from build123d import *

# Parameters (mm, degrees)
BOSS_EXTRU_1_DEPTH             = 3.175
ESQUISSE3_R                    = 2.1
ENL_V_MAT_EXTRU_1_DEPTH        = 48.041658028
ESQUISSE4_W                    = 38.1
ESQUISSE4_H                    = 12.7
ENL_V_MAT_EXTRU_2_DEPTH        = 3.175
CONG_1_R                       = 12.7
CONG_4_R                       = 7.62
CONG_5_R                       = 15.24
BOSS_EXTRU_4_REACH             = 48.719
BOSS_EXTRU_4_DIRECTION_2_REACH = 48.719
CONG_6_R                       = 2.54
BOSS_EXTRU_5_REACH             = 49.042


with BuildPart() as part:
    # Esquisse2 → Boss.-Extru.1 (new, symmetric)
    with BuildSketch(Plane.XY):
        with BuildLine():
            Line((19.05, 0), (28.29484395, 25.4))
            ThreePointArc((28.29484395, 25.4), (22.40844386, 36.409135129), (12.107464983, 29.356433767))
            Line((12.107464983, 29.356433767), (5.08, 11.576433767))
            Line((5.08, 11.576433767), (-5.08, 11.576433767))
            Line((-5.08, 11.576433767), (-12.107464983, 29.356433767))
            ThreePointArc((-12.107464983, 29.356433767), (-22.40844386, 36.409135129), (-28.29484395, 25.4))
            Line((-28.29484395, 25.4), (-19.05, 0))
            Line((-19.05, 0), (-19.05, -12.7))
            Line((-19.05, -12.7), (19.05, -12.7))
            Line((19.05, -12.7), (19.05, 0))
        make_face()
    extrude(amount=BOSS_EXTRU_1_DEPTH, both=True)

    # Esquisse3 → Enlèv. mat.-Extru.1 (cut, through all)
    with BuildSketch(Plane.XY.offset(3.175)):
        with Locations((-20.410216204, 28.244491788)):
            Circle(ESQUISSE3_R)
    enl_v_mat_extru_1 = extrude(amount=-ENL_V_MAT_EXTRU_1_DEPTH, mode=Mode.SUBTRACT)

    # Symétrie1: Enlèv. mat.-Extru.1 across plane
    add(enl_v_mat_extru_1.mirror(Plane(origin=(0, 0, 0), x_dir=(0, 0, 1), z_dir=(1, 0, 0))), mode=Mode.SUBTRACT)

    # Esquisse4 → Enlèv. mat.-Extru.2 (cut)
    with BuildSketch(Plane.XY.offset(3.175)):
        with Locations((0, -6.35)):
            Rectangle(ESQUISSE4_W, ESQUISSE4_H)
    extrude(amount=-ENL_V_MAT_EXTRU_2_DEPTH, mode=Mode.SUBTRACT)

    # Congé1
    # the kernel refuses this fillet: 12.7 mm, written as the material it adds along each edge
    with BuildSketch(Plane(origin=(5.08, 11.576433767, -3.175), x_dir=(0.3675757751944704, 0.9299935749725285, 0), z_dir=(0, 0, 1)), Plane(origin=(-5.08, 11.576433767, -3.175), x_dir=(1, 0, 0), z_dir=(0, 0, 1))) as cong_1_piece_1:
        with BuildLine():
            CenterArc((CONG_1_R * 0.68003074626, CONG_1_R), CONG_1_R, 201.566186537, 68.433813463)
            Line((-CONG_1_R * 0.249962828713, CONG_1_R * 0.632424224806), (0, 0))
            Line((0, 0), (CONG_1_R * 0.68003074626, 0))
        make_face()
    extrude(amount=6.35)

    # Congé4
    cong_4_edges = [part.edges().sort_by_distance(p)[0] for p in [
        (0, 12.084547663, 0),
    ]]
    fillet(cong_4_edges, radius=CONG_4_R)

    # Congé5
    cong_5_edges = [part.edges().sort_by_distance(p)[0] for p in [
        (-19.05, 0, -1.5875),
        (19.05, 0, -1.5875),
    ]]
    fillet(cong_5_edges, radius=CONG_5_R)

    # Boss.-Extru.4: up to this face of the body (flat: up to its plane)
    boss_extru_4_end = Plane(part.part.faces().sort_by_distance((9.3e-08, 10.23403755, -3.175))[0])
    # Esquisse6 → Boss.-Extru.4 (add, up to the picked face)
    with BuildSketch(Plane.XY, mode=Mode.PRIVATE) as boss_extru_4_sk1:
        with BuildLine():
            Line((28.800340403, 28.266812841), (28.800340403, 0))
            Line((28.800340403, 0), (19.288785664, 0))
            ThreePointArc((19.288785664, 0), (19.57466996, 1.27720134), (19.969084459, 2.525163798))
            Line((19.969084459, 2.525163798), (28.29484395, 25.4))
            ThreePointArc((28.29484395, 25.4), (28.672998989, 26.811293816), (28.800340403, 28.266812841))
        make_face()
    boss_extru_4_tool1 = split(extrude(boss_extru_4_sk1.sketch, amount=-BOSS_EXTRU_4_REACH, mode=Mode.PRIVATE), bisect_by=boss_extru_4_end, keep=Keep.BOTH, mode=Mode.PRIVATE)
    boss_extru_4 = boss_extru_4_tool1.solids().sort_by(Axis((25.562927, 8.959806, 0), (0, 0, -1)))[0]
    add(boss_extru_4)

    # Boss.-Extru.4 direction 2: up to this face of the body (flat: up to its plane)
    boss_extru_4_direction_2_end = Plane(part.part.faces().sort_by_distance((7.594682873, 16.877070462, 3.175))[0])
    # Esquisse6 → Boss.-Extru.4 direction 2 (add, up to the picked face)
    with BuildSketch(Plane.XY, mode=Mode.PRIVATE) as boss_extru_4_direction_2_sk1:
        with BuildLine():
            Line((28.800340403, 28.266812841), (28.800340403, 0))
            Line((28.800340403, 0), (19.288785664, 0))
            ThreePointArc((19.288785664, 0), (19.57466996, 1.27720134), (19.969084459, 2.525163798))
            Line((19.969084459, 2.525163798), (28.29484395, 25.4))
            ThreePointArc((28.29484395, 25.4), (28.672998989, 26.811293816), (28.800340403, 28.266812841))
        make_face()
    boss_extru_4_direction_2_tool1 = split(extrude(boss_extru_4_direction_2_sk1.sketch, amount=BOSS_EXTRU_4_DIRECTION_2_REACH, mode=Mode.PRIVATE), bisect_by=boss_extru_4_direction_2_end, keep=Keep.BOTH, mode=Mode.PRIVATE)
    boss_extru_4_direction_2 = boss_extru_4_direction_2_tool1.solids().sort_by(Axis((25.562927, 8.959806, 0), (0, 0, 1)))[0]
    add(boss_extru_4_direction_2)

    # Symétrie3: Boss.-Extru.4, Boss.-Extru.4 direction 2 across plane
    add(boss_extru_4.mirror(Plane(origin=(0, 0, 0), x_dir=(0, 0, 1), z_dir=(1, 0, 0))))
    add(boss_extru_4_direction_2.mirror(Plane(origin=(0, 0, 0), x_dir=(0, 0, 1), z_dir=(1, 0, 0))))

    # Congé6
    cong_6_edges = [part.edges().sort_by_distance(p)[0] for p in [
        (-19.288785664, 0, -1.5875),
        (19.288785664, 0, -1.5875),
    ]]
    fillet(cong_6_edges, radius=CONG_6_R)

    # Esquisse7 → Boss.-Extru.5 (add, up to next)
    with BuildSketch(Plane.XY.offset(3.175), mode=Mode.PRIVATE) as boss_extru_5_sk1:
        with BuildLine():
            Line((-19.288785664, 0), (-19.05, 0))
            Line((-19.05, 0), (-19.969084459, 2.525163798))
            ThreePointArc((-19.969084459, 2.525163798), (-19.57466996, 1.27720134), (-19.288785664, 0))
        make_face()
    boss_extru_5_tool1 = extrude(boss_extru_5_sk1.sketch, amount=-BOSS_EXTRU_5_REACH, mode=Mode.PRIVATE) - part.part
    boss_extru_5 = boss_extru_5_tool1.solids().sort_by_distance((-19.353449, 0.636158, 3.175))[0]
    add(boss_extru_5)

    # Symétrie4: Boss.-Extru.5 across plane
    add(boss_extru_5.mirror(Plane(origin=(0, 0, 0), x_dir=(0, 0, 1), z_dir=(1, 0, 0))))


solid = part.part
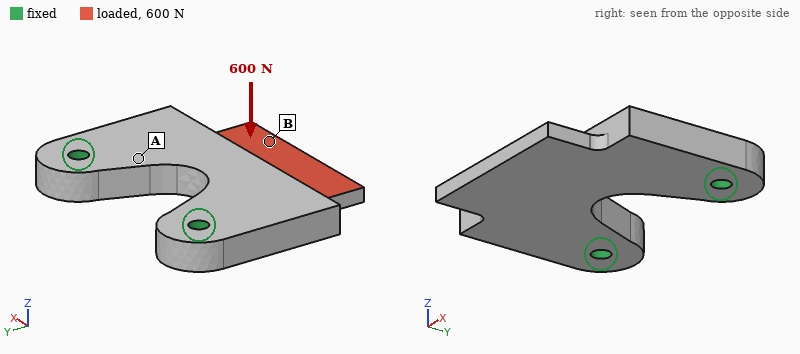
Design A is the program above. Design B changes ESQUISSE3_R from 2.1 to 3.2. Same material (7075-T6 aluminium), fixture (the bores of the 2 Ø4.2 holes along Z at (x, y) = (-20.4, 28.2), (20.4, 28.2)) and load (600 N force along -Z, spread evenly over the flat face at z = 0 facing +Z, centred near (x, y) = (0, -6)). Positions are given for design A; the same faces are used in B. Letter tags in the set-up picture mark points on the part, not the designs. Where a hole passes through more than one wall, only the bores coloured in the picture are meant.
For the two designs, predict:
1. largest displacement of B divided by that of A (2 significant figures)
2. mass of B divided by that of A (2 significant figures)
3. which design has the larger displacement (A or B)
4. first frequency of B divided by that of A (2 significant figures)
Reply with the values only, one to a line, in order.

0.88
0.98
A
1.1
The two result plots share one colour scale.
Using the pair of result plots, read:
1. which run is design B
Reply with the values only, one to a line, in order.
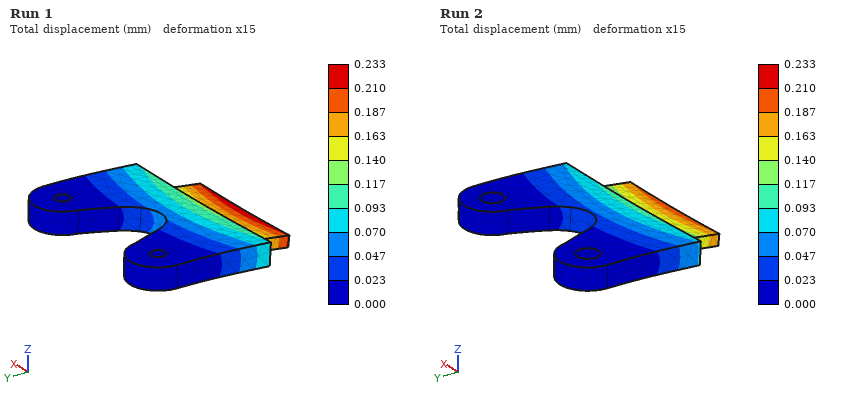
Run 2
